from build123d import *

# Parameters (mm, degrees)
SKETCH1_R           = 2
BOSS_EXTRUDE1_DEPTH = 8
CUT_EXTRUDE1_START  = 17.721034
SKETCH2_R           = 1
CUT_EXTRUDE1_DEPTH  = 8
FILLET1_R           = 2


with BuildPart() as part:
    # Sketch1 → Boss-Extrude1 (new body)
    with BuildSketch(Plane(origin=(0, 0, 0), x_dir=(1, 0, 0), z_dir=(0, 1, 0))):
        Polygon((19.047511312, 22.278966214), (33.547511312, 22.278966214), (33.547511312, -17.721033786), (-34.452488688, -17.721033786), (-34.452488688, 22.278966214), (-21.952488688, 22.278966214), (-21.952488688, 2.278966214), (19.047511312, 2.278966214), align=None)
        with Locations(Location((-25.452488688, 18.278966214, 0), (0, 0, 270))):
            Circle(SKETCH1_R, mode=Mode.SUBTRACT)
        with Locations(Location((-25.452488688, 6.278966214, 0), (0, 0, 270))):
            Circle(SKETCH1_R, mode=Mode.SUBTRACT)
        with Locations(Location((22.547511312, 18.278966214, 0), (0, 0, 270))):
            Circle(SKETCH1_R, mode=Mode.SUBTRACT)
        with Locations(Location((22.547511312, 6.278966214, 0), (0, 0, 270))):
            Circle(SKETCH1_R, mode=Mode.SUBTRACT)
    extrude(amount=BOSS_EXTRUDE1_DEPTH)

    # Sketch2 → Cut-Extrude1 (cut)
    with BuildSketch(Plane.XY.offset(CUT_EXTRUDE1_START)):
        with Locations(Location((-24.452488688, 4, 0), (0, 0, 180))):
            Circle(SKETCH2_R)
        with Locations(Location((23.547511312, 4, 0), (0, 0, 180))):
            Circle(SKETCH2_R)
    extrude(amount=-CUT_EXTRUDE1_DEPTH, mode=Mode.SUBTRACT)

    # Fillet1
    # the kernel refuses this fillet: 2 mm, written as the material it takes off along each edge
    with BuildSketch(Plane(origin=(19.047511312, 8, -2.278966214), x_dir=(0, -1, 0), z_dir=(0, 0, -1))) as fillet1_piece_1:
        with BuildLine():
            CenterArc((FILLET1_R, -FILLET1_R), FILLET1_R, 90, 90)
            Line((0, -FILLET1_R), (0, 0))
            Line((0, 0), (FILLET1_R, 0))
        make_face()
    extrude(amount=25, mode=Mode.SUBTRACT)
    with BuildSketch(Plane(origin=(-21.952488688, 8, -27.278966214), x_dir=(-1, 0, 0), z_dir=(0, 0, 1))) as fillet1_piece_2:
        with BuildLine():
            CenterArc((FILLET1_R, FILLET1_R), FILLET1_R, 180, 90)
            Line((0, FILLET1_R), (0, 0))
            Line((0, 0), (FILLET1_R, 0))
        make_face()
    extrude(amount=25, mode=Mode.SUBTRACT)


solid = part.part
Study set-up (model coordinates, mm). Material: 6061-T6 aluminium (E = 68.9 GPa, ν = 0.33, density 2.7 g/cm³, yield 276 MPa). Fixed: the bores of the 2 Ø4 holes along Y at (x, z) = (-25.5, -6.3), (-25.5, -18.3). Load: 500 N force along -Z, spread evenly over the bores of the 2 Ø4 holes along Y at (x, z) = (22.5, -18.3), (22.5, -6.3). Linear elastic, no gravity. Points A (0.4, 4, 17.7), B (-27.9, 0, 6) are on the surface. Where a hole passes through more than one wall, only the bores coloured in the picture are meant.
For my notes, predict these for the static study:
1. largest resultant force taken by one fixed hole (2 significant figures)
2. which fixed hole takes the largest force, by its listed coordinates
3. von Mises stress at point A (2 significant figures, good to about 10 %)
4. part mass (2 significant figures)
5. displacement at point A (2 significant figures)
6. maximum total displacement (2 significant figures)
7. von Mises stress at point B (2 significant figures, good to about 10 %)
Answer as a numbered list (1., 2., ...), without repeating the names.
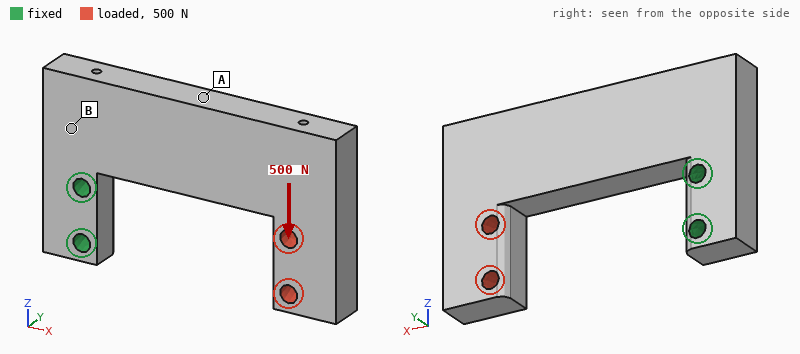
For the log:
1. 1.9 kN
2. (-25.5, -6.3)
3. 21 MPa
4. 40 g
5. 0.15 mm
6. 0.31 mm
7. 41 MPa
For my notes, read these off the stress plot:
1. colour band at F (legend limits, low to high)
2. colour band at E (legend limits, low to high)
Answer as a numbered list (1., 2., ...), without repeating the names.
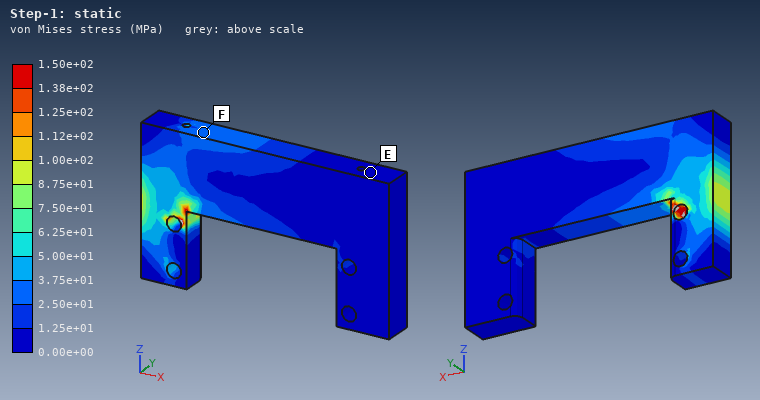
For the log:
1. 2.50e+01 to 3.75e+01 MPa
2. 0.00e+00 to 1.25e+01 MPa
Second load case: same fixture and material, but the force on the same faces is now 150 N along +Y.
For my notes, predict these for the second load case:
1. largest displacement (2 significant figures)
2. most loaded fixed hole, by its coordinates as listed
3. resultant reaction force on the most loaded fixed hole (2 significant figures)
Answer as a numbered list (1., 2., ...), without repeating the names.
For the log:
1. 0.31 mm
2. (-25.5, -6.3)
3. 120 N
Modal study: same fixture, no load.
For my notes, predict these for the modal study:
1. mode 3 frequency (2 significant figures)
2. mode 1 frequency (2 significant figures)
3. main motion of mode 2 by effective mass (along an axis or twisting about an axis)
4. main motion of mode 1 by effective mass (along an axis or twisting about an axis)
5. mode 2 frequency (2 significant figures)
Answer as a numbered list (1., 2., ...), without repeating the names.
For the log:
1. 3100 Hz
2. 1000 Hz
3. along Z
4. along Y
5. 1600 Hz
